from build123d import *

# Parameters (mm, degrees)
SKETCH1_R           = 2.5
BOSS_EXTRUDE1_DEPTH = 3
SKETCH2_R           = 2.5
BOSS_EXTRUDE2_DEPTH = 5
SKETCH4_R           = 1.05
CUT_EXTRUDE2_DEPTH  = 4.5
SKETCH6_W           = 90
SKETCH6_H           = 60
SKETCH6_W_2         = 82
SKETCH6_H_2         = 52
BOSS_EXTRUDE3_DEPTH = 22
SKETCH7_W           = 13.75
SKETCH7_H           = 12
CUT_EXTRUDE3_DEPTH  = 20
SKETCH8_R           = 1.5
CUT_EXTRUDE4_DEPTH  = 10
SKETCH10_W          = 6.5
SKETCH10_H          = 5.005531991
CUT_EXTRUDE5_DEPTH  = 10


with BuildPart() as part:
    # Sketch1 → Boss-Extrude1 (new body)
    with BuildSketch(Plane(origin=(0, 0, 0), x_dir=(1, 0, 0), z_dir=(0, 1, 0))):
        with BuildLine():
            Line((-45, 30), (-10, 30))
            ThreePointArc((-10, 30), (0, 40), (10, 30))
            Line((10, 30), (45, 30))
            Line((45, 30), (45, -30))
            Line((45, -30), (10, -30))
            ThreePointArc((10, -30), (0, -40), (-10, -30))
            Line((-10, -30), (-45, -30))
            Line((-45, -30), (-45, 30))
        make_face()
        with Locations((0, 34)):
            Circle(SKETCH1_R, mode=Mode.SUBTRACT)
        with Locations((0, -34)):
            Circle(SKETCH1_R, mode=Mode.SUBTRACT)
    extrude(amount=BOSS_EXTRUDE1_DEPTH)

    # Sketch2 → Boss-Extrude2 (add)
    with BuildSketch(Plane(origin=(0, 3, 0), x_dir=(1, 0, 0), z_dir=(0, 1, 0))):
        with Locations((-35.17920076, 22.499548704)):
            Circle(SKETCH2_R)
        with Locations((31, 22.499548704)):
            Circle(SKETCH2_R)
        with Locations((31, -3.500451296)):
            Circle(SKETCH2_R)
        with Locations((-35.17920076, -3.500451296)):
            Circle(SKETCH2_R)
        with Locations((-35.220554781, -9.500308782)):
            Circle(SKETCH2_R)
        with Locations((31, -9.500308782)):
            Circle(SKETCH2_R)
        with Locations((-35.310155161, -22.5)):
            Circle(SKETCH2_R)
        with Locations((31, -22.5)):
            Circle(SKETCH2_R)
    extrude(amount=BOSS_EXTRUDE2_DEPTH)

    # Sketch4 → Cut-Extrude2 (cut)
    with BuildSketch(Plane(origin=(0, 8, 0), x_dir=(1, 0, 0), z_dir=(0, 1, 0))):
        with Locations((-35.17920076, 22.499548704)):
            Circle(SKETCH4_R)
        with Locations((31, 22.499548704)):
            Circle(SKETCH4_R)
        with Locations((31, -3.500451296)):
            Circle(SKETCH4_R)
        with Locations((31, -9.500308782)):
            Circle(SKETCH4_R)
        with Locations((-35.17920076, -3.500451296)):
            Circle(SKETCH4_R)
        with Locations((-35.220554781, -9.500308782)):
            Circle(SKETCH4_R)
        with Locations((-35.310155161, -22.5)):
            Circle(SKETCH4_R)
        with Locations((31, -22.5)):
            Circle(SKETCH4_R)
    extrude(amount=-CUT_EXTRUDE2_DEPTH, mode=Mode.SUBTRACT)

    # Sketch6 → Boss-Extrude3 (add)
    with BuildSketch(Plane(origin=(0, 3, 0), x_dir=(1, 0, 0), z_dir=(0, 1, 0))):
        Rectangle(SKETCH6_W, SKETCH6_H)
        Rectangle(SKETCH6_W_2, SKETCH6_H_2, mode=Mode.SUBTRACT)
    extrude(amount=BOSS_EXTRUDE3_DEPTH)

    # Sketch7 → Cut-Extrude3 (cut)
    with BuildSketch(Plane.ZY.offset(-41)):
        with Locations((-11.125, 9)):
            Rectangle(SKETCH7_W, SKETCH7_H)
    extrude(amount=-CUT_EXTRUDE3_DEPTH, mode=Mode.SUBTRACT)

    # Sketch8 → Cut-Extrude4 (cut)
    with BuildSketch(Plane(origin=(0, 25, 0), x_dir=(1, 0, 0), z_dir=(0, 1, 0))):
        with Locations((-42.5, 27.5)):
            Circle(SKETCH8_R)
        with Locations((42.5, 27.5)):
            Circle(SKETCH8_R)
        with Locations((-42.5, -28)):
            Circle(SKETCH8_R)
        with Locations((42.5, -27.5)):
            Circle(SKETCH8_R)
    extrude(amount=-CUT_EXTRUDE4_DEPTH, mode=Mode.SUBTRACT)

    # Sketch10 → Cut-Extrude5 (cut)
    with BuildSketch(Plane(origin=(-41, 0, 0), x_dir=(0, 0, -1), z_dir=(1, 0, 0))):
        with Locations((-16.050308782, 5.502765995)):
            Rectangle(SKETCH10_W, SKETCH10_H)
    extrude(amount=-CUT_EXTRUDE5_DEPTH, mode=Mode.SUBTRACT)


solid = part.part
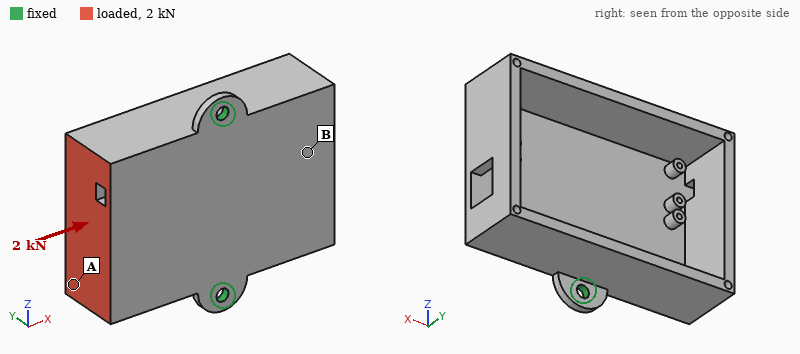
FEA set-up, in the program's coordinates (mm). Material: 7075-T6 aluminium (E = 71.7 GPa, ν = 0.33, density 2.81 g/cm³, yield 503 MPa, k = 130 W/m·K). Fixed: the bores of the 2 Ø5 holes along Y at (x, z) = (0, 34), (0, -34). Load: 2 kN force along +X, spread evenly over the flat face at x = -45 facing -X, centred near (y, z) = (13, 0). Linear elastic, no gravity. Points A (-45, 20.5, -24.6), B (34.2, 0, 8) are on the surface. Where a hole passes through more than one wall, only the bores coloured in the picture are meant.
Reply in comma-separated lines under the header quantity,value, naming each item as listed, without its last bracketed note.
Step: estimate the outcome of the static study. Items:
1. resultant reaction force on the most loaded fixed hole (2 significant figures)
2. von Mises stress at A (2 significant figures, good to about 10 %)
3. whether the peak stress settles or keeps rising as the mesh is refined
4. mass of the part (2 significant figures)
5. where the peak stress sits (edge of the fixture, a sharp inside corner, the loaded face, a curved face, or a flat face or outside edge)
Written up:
quantity,value
resultant reaction force on the most loaded fixed hole,1.0 kN
von Mises stress at A,46 MPa
whether the peak stress settles or keeps rising as the mesh is refined,keeps rising
mass of the part,120 g
where the peak stress sits,edge of the fixture
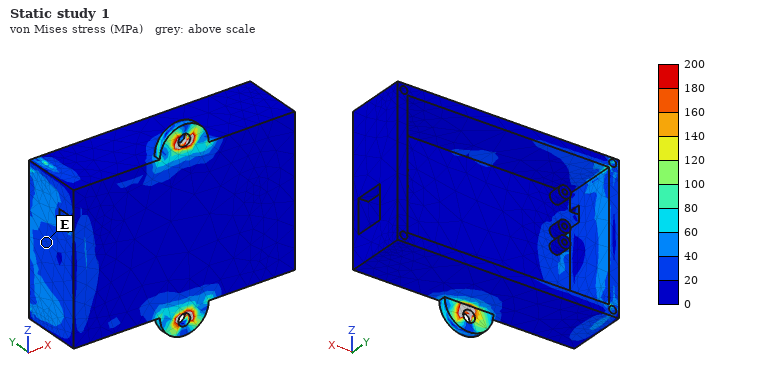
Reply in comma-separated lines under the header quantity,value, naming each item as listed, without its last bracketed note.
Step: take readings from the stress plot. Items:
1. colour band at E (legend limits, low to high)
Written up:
quantity,value
colour band at E,20 to 40 MPa
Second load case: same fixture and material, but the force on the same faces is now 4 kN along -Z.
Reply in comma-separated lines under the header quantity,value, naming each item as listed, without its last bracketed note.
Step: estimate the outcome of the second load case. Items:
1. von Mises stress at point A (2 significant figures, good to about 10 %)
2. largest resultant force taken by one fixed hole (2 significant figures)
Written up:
quantity,value
von Mises stress at point A,70 MPa
largest resultant force taken by one fixed hole,3.4 kN
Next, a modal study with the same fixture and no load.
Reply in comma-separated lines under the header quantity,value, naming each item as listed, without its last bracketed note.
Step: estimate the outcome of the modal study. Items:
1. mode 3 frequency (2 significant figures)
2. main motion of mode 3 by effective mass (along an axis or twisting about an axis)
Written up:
quantity,value
mode 3 frequency,3300 Hz
main motion of mode 3 by effective mass,along Y
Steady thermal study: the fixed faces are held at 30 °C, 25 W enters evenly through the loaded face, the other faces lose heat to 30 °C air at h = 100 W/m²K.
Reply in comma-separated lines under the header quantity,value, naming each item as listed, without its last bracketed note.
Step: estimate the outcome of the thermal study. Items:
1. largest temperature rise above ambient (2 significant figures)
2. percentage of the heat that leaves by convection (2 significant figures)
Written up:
quantity,value
largest temperature rise above ambient,24 K
percentage of the heat that leaves by convection,67 %
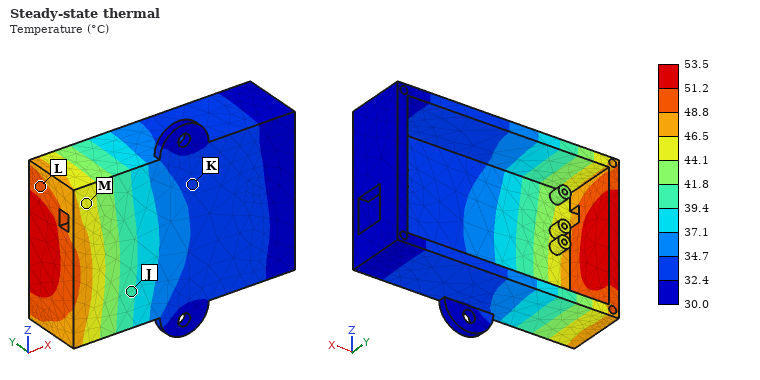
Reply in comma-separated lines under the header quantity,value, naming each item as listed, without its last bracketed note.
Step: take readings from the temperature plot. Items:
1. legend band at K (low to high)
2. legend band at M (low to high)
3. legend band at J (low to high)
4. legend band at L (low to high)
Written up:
quantity,value
legend band at K,32.4 to 34.7 °C
legend band at M,44.1 to 46.5 °C
legend band at J,39.4 to 41.8 °C
legend band at L,48.8 to 51.2 °C
